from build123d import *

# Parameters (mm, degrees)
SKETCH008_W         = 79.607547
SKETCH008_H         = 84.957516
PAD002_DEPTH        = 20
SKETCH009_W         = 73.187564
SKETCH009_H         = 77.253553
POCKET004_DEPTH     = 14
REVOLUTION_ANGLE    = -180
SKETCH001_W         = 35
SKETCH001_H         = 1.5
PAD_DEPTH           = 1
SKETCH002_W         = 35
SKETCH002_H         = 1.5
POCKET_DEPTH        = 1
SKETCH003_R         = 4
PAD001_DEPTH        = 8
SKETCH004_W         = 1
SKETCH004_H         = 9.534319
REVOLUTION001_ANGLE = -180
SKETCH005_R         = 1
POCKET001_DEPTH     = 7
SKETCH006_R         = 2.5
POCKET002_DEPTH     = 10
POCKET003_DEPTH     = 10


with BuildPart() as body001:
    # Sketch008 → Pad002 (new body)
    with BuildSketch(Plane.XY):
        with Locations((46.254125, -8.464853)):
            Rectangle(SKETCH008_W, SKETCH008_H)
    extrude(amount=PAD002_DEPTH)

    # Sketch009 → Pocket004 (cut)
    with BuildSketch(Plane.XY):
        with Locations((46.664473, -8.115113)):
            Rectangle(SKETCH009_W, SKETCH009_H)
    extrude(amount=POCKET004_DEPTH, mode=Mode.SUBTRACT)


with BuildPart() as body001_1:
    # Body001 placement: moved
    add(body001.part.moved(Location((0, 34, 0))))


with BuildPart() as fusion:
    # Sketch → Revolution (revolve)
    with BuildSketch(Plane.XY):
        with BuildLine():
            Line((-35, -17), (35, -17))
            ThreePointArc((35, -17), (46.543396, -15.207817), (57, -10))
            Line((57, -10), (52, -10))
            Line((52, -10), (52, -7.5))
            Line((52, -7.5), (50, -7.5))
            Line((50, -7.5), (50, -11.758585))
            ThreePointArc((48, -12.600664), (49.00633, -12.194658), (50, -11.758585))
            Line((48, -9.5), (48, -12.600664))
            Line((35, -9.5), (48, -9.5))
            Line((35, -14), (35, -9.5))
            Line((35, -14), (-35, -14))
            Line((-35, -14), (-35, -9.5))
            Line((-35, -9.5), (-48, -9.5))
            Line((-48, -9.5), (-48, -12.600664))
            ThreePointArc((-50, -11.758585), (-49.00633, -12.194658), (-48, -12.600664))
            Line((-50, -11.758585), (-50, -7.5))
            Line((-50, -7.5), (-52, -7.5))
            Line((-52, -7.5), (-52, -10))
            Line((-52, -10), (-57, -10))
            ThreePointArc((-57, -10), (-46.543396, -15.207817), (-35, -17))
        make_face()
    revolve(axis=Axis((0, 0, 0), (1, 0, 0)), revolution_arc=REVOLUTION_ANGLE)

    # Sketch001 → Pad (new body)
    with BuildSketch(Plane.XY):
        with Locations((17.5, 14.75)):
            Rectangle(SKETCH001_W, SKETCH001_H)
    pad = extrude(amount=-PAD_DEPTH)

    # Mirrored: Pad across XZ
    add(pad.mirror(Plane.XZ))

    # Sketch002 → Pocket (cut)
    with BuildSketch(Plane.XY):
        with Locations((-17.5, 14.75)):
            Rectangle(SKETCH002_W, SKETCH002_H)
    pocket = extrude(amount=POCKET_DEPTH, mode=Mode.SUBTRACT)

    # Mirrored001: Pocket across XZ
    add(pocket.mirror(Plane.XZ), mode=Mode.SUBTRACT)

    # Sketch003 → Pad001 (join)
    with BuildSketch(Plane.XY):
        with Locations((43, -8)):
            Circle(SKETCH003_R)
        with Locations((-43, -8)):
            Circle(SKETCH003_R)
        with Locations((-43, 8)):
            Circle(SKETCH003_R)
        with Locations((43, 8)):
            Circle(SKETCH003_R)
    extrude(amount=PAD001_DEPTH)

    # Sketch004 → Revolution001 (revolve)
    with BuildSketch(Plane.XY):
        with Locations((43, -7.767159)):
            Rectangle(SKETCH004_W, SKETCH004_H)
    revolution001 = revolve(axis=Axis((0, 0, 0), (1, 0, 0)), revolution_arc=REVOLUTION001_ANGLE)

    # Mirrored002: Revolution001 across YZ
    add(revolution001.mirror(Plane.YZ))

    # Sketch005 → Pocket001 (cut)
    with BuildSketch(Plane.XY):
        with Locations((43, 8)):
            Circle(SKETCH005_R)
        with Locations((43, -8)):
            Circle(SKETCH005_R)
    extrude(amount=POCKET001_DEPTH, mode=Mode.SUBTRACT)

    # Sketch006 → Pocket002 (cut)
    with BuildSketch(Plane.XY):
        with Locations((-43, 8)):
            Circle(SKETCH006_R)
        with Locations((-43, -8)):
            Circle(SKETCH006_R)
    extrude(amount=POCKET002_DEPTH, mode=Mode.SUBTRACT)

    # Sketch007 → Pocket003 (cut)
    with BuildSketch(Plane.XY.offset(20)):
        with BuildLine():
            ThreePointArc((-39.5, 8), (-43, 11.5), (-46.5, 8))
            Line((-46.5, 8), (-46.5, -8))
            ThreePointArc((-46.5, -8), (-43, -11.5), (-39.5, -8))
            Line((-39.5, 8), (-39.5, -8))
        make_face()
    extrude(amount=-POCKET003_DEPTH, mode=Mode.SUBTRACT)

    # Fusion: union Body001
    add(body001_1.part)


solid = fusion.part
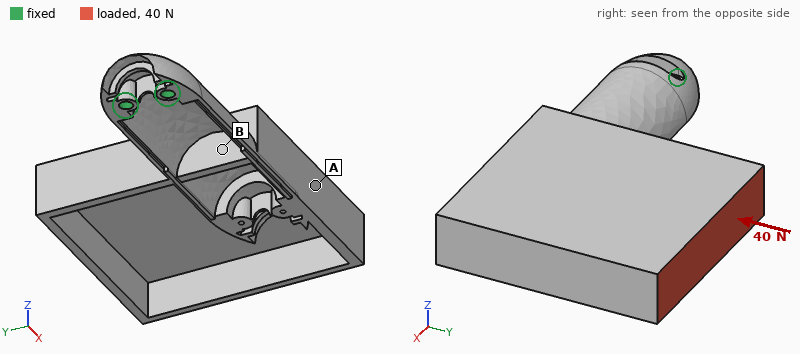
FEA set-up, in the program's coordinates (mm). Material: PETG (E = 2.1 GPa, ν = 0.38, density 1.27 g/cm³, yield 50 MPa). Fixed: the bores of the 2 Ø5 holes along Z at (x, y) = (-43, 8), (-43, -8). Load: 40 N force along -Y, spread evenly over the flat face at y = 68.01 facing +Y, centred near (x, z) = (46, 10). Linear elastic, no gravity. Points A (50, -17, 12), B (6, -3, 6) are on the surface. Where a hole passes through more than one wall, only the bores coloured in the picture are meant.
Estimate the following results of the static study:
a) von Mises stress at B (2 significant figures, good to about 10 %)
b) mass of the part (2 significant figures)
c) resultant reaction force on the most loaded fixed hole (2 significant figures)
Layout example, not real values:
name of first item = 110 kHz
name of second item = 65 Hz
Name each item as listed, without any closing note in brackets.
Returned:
von Mises stress at B = 1.2 MPa
mass of the part = 92 g
resultant reaction force on the most loaded fixed hole = 150 N
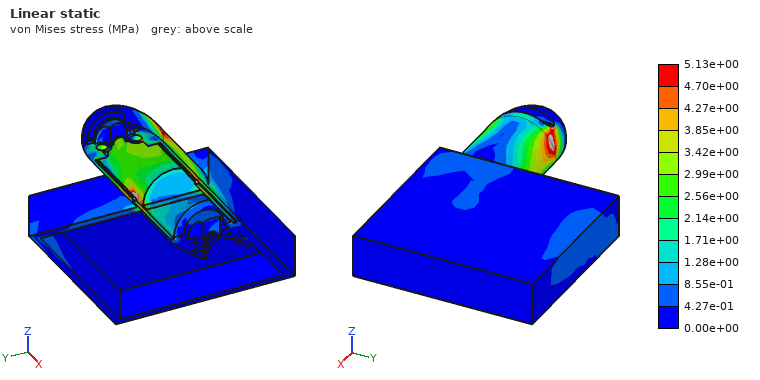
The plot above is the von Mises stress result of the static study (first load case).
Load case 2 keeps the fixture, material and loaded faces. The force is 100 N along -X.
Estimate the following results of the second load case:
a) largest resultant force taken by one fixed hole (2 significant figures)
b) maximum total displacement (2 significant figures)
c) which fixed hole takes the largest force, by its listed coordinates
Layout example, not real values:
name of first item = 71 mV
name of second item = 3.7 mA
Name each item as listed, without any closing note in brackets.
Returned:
largest resultant force taken by one fixed hole = 340 N
maximum total displacement = 2.0 mm
which fixed hole takes the largest force, by its listed coordinates = (-43, 8)
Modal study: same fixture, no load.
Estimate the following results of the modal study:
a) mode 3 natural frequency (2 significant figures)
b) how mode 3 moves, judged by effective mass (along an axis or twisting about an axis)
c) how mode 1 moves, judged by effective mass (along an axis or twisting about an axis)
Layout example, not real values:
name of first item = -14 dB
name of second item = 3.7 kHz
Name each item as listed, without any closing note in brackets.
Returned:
mode 3 natural frequency = 170 Hz
how mode 3 moves, judged by effective mass = along Y
how mode 1 moves, judged by effective mass = along Z
